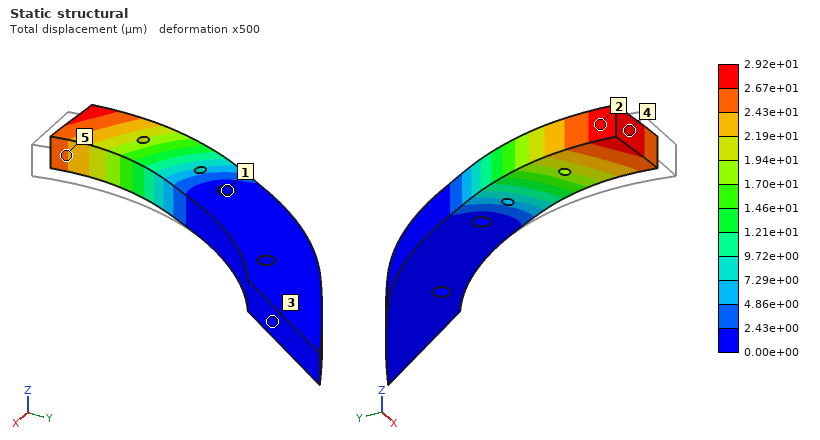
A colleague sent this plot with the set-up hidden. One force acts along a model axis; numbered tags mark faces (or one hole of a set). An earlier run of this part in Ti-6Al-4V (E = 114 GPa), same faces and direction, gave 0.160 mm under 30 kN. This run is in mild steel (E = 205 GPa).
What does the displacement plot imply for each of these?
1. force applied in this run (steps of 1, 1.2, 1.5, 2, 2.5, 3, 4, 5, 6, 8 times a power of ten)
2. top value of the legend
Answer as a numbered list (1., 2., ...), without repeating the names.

1. 10 kN
2. 2.92e+01 µm
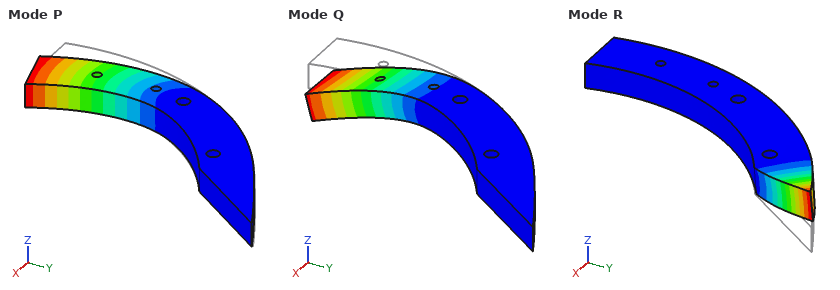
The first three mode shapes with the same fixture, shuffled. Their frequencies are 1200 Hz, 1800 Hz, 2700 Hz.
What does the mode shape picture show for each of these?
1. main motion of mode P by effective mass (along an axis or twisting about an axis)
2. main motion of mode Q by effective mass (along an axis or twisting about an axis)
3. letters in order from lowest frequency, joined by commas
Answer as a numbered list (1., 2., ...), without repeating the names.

1. along X
2. along Z
3. Q, P, R
